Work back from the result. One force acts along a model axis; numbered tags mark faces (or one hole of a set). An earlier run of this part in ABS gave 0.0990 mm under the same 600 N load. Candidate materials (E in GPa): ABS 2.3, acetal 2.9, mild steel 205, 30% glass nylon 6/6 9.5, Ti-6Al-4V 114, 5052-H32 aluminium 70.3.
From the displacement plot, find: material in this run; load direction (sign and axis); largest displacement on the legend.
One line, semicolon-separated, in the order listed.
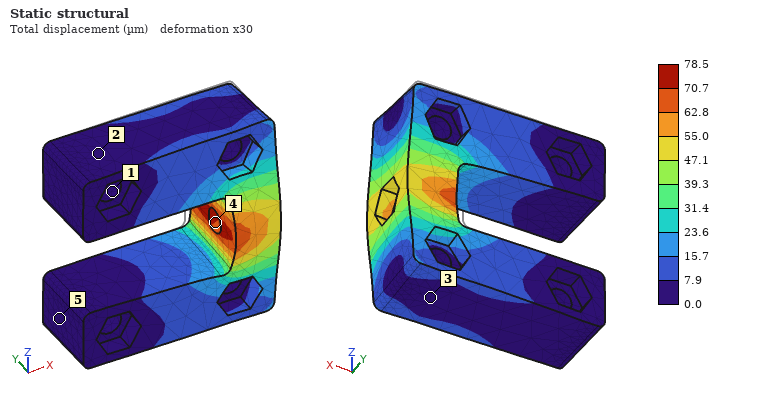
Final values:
acetal; -Y; 78.5 µm
